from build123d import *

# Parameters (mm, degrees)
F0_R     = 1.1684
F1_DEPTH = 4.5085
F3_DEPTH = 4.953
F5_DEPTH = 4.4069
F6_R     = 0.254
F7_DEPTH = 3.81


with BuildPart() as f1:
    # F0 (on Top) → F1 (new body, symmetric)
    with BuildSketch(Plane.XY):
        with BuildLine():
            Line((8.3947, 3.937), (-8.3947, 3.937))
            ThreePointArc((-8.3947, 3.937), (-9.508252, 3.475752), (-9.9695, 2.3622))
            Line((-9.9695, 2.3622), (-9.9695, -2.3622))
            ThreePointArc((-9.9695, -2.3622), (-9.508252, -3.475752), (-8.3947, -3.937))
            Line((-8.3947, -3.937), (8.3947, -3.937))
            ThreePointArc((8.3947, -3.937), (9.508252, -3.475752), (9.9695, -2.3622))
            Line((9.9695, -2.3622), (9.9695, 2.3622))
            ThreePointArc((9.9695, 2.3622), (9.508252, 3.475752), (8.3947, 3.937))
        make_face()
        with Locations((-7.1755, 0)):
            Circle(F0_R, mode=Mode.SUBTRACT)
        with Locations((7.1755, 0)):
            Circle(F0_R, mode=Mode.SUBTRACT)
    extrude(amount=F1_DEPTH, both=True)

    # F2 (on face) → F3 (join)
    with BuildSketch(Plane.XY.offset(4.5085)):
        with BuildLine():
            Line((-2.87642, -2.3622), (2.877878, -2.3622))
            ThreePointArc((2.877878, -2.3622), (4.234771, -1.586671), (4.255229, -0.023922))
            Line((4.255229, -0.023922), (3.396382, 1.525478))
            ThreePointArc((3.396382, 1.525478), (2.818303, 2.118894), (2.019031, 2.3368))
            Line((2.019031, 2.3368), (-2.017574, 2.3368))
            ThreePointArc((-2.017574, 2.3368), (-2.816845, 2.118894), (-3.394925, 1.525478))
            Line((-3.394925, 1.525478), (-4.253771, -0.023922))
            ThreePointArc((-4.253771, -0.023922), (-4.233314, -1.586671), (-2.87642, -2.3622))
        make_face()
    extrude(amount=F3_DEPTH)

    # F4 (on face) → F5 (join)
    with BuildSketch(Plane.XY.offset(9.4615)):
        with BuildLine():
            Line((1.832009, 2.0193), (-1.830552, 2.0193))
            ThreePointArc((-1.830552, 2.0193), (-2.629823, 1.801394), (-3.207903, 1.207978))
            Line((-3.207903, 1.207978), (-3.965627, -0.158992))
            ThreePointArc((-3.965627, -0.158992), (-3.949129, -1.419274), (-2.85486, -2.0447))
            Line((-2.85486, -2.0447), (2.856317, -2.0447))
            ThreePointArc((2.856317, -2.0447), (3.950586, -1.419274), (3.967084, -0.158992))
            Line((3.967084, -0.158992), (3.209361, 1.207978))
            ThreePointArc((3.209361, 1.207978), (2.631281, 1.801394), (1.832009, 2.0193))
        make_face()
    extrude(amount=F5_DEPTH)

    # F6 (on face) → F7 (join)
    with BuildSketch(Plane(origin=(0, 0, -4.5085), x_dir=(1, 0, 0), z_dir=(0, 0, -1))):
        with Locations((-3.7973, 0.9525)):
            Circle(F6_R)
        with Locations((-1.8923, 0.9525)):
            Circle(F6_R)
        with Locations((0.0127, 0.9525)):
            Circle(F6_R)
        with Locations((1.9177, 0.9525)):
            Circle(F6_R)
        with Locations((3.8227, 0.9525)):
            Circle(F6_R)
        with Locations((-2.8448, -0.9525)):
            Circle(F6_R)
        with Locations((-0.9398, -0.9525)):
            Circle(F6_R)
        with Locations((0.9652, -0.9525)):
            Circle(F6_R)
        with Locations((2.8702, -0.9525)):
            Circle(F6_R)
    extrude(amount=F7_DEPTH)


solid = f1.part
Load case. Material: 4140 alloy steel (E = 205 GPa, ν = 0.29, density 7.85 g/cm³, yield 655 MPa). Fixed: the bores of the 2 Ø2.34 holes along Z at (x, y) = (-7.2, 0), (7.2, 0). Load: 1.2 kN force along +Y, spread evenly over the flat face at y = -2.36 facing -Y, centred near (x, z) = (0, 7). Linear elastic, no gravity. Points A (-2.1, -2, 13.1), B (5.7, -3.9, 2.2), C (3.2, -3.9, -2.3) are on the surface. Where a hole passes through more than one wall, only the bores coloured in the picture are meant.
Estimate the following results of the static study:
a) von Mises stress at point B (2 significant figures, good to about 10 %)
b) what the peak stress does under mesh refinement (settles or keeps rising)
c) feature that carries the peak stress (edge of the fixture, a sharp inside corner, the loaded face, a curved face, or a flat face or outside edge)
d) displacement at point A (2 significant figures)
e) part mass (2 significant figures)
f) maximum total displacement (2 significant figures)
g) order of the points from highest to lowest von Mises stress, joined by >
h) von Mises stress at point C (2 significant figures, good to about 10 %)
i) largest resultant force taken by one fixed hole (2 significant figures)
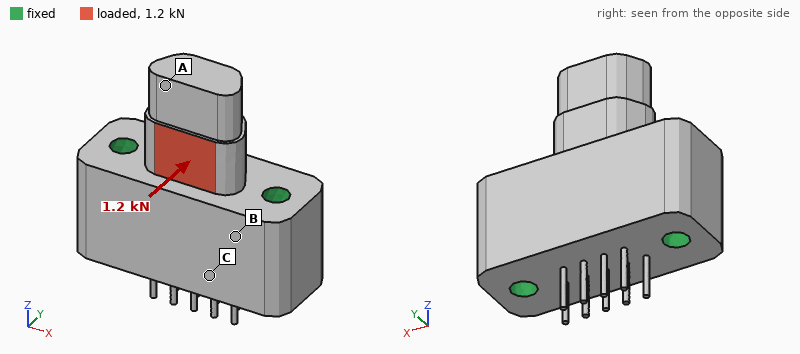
46 MPa
keeps rising
edge of the fixture
13 µm
13 g
14 µm
B > C > A
27 MPa
600 N
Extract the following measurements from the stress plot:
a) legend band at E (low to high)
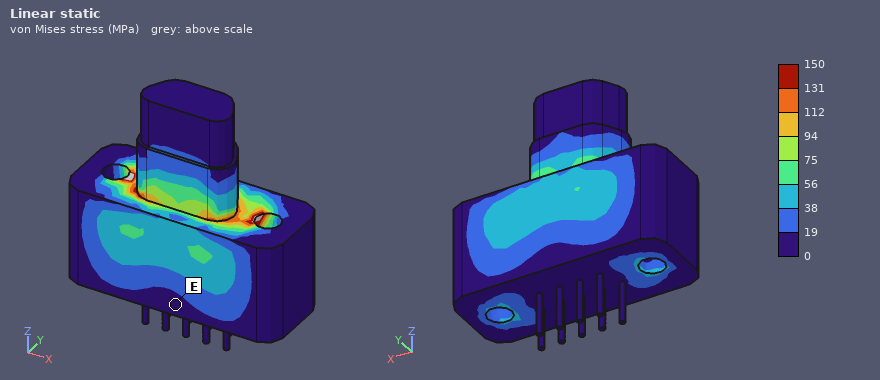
0 to 19 MPa
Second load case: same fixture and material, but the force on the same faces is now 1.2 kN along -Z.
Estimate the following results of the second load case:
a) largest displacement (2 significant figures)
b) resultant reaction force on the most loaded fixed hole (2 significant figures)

8.7 µm
620 N
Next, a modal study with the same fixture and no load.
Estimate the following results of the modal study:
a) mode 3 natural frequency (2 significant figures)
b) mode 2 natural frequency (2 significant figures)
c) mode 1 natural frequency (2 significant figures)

23 kHz
23 kHz
23 kHz
